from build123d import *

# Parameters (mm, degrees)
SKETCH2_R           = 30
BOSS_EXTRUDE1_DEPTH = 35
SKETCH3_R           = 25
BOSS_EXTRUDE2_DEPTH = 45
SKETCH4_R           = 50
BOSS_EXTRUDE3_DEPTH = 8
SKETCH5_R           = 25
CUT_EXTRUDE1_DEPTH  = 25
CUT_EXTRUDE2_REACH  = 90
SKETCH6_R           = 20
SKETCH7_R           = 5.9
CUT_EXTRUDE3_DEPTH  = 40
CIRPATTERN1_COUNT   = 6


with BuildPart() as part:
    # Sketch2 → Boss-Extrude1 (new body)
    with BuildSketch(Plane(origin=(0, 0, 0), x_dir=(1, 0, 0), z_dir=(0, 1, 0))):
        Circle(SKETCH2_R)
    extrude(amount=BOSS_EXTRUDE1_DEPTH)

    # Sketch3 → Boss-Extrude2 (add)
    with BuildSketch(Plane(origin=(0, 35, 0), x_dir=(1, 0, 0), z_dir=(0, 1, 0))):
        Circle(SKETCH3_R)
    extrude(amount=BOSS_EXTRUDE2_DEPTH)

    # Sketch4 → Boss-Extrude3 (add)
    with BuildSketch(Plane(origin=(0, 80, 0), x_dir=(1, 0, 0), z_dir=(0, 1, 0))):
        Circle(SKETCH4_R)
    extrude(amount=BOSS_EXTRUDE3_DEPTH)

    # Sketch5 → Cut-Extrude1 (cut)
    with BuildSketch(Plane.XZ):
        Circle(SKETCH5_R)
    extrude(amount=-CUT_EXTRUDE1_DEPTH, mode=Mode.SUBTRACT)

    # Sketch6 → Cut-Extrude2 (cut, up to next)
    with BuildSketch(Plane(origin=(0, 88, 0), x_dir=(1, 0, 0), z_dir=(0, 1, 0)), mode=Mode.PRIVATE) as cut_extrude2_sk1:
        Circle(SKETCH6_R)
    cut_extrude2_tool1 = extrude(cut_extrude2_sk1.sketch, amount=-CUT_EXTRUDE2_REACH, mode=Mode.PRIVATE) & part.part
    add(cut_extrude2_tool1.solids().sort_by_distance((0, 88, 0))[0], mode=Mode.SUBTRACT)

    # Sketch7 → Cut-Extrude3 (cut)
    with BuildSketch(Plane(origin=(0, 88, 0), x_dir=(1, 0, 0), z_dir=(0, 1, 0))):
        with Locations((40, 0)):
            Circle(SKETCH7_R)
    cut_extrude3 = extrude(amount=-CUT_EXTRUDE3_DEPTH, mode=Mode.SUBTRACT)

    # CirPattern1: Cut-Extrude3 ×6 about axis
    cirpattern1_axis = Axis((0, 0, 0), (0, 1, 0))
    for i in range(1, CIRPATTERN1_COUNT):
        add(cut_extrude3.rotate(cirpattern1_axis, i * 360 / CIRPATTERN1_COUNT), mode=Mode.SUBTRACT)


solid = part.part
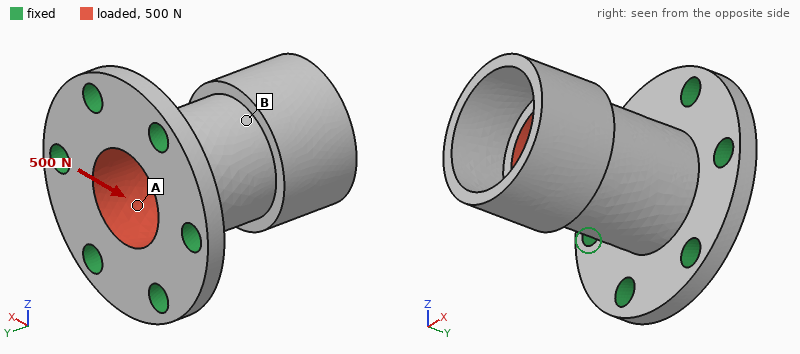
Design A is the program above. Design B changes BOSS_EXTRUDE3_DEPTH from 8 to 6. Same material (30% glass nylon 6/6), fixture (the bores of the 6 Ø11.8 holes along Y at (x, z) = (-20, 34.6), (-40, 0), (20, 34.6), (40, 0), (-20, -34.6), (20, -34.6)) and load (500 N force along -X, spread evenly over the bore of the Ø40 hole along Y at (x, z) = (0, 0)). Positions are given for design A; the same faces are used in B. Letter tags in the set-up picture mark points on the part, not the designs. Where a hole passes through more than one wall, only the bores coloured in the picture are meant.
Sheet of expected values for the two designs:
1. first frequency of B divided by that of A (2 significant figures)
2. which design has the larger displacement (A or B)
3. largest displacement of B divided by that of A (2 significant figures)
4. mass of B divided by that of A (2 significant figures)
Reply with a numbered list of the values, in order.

1. 0.87
2. B
3. 1.4
4. 0.90
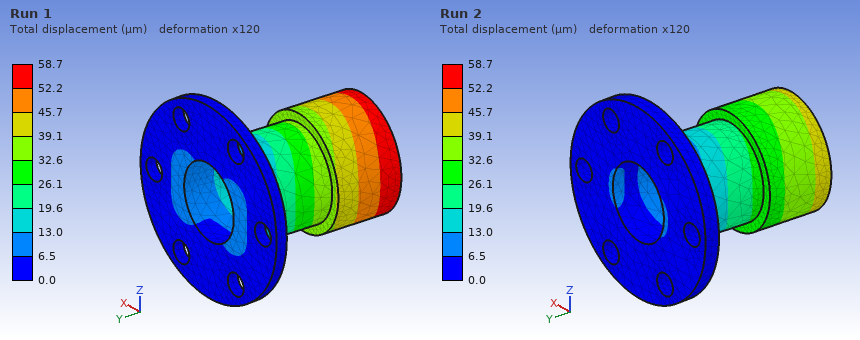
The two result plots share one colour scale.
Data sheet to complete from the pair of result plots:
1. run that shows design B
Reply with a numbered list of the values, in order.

1. Run 1
